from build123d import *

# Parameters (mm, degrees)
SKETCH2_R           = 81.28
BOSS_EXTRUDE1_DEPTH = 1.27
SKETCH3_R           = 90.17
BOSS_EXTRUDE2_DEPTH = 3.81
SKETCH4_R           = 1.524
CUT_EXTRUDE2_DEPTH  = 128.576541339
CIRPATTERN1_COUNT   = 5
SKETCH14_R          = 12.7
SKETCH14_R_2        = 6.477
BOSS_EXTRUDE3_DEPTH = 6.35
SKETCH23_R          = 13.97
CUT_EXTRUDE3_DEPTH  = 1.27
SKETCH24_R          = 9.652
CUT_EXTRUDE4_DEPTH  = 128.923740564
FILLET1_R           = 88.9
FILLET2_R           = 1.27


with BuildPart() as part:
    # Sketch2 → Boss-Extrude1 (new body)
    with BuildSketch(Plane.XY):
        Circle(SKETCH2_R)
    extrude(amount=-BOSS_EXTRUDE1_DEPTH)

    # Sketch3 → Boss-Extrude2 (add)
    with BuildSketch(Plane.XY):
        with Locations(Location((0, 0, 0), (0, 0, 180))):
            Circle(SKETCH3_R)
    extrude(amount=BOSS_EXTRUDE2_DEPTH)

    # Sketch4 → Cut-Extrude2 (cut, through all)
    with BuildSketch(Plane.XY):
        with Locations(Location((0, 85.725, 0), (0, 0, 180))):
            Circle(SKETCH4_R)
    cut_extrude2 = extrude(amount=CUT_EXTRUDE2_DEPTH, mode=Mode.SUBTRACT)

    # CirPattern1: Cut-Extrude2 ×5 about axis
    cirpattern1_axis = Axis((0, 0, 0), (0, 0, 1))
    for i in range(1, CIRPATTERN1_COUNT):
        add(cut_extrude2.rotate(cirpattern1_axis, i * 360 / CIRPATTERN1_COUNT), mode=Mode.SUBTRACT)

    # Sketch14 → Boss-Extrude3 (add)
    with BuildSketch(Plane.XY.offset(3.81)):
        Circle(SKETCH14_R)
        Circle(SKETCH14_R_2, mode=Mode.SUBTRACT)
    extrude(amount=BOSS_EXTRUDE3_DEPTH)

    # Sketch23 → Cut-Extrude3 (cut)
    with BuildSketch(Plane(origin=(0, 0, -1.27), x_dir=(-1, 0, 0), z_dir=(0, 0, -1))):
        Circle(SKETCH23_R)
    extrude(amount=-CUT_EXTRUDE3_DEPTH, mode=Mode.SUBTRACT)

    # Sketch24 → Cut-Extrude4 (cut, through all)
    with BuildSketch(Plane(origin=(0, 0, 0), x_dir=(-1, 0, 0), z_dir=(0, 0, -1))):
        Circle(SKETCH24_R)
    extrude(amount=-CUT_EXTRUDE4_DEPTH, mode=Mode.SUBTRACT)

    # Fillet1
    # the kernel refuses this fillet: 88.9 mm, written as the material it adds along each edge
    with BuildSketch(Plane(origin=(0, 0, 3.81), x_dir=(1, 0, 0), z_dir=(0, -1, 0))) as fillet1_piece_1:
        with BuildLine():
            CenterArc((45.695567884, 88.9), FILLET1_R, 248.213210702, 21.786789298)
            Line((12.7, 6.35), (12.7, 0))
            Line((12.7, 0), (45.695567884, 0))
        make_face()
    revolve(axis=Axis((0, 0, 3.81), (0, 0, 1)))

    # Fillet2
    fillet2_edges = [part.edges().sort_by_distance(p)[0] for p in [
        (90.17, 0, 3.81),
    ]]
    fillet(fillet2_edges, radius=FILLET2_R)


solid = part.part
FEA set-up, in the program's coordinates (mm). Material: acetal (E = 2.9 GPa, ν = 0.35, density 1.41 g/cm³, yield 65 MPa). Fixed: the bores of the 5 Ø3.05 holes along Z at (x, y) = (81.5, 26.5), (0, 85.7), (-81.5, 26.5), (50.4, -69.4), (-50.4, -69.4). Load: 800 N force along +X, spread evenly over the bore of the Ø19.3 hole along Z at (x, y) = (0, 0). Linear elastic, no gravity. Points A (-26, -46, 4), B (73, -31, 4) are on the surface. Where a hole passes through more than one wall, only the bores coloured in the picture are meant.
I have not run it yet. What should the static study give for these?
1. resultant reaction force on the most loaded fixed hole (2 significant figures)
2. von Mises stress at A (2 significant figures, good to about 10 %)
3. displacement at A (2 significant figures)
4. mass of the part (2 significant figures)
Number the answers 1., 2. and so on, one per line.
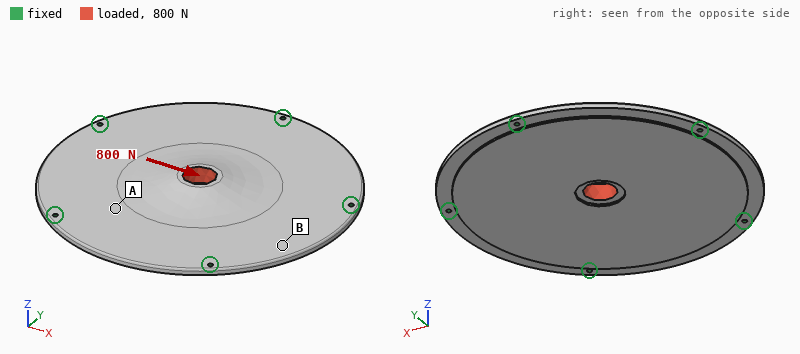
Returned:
1. 200 N
2. 1.5 MPa
3. 0.054 mm
4. 190 g
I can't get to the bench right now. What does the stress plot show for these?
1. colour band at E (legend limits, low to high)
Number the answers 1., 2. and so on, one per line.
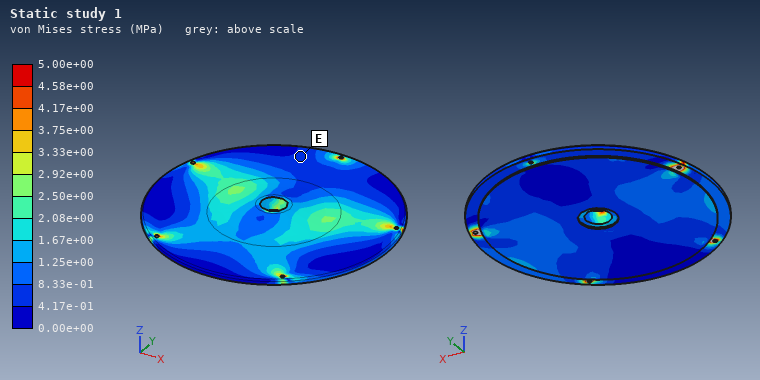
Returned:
1. 4.17e-01 to 8.33e-01 MPa
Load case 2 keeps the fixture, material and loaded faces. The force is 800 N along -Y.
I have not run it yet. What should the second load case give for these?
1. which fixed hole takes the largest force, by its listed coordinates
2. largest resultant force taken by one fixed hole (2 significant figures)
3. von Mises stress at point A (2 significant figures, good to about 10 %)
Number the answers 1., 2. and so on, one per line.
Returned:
1. (0, 85.7)
2. 200 N
3. 1.8 MPa
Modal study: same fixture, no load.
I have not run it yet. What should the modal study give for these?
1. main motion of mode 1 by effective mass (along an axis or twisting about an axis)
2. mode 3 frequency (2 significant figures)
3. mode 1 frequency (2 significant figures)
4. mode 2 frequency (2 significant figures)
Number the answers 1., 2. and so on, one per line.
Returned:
1. along Z
2. 550 Hz
3. 320 Hz
4. 550 Hz
